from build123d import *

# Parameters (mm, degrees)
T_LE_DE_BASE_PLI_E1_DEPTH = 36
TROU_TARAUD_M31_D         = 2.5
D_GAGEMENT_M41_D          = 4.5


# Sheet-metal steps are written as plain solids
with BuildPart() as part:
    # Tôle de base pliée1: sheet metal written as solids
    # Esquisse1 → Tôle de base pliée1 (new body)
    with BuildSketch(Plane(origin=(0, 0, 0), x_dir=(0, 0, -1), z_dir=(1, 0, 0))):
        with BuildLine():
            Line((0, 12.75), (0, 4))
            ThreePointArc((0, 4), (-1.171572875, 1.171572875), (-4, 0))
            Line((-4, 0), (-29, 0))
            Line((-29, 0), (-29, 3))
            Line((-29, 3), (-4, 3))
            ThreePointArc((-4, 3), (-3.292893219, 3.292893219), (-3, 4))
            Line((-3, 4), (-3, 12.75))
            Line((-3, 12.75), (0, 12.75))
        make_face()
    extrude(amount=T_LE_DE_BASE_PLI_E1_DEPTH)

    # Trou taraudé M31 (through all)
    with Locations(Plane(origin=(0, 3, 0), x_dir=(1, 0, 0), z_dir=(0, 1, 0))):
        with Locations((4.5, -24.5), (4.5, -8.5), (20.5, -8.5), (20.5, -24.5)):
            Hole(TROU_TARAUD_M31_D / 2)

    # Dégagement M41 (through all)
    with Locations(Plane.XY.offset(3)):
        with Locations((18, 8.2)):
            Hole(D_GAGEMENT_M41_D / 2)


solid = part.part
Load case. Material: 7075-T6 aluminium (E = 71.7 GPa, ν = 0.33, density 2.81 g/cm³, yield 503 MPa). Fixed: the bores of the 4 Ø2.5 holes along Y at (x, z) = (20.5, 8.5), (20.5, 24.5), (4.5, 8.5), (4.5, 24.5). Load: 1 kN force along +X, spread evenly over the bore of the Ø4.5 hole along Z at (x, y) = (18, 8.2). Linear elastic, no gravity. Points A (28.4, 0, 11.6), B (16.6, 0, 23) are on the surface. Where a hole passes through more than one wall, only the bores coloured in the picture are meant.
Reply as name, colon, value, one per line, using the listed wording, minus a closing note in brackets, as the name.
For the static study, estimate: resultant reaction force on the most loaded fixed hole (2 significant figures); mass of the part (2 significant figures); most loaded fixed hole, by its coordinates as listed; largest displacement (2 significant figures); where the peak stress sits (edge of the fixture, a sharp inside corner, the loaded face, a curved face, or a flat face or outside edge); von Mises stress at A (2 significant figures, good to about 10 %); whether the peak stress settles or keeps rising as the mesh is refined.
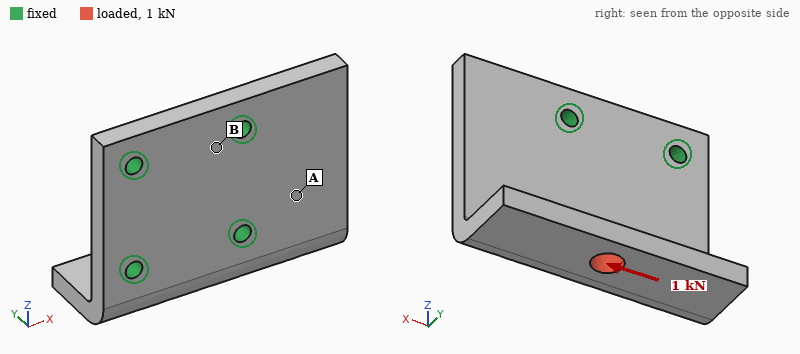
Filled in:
resultant reaction force on the most loaded fixed hole: 760 N
mass of the part: 11 g
most loaded fixed hole, by its coordinates as listed: (20.5, 8.5)
largest displacement: 53 µm
where the peak stress sits: edge of the fixture
von Mises stress at A: 26 MPa
whether the peak stress settles or keeps rising as the mesh is refined: keeps rising
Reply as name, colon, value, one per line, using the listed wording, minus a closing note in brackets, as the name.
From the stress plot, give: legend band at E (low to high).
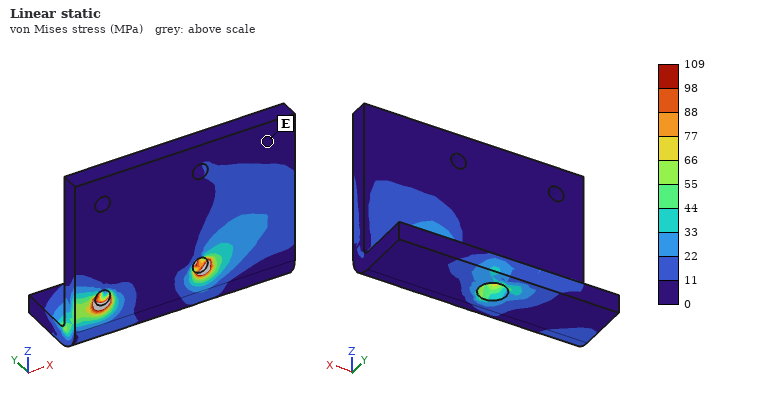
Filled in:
legend band at E: 0 to 11 MPa
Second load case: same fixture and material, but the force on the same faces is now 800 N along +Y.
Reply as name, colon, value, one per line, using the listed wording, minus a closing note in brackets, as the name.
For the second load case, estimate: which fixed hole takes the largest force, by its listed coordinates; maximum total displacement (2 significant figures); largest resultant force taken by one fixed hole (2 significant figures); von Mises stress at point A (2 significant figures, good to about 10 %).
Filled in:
which fixed hole takes the largest force, by its listed coordinates: (20.5, 8.5)
maximum total displacement: 66 µm
largest resultant force taken by one fixed hole: 720 N
von Mises stress at point A: 34 MPa
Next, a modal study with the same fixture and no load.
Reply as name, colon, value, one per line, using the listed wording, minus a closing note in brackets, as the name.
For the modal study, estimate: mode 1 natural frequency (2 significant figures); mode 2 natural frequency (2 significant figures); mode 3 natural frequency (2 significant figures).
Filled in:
mode 1 natural frequency: 8800 Hz
mode 2 natural frequency: 11 kHz
mode 3 natural frequency: 12 kHz
